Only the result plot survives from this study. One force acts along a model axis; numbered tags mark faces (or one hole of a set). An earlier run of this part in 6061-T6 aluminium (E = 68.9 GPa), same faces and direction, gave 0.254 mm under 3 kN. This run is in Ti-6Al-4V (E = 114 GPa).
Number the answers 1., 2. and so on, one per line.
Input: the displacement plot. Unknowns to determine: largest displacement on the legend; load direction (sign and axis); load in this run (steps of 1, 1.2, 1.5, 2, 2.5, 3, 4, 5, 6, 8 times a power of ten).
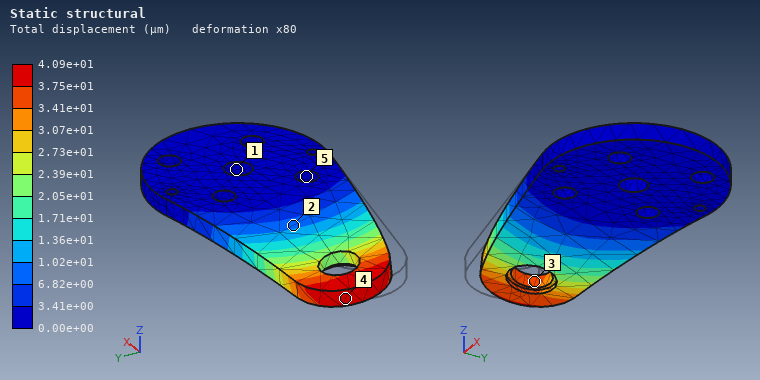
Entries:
1. 4.09e+01 µm
2. +Y
3. 800 N
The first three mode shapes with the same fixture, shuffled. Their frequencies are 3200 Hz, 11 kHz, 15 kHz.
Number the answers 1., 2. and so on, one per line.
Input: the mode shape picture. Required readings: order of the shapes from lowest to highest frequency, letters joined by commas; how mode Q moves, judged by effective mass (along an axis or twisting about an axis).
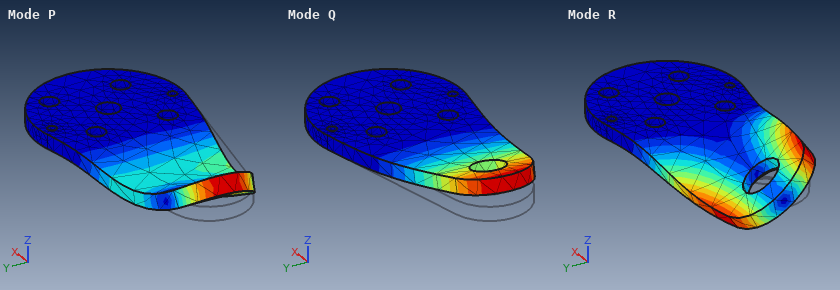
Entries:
1. Q, R, P
2. along Z
